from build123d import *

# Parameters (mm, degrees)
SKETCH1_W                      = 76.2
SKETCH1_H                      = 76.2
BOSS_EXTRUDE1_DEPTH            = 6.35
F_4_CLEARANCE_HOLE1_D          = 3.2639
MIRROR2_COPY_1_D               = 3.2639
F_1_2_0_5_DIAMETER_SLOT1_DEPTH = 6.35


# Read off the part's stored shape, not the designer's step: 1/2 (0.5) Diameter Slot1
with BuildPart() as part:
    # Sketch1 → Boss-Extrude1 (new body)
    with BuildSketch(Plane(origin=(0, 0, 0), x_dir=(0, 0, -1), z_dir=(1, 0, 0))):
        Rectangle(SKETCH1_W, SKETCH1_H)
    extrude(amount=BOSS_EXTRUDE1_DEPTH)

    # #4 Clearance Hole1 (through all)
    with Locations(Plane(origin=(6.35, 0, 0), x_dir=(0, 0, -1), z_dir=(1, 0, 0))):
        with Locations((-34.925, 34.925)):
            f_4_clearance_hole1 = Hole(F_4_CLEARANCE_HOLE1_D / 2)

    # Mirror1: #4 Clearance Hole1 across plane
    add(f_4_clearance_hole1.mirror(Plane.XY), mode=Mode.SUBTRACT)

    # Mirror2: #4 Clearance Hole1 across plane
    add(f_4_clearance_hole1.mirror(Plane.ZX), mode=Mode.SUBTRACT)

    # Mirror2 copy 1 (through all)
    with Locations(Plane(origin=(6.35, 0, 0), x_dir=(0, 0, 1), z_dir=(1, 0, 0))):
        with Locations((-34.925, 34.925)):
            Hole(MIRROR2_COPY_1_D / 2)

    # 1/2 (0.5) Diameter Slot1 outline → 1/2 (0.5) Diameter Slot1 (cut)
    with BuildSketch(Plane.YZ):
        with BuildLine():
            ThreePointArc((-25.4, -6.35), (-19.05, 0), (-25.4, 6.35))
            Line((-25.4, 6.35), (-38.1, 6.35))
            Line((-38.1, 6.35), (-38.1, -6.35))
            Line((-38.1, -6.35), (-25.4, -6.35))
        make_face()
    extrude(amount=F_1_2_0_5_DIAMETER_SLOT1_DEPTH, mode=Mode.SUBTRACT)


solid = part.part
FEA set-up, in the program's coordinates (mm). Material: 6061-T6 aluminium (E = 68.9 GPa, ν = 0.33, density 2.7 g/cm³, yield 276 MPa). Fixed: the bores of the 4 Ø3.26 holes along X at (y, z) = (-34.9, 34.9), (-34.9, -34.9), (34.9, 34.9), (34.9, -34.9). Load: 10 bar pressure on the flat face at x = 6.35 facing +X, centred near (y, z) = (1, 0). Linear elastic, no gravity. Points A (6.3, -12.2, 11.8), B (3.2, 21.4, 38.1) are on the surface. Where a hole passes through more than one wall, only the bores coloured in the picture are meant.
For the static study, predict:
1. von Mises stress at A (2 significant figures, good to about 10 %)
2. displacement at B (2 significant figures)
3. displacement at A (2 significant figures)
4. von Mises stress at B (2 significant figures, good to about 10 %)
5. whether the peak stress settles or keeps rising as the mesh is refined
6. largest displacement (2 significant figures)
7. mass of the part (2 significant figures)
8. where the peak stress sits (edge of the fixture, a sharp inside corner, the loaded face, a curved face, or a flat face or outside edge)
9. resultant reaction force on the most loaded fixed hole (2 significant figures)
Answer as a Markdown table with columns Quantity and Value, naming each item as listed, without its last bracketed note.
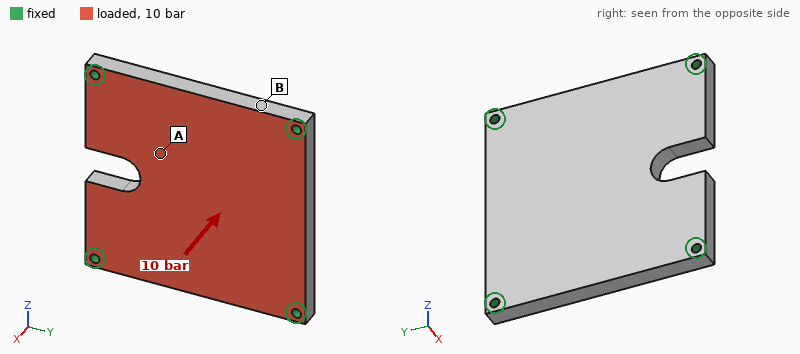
| Quantity | Value |
|---|---|
| von Mises stress at A | 43 MPa |
| displacement at B | 0.028 mm |
| displacement at A | 0.14 mm |
| von Mises stress at B | 22 MPa |
| whether the peak stress settles or keeps rising as the mesh is refined | keeps rising |
| largest displacement | 0.15 mm |
| mass of the part | 95 g |
| where the peak stress sits | edge of the fixture |
| resultant reaction force on the most loaded fixed hole | 1.4 kN |
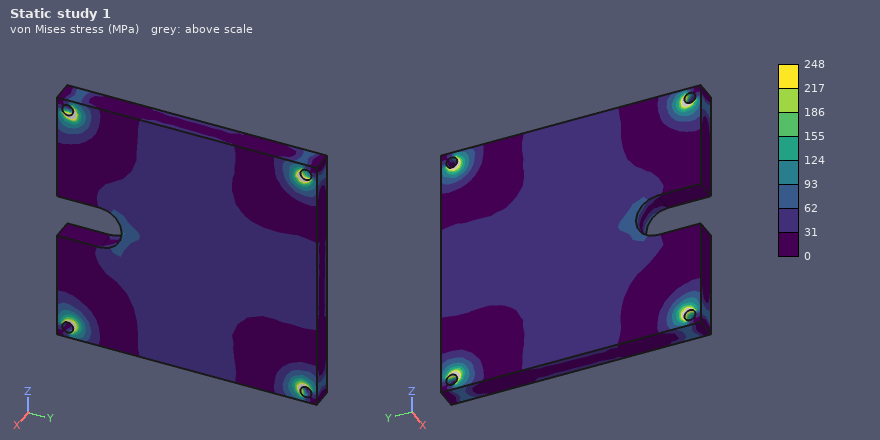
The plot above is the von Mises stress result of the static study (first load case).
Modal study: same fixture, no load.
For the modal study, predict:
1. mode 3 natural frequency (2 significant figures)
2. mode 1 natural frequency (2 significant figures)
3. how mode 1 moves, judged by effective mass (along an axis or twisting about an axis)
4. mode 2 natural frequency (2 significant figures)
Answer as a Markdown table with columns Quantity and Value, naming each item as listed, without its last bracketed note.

| Quantity | Value |
|---|---|
| mode 3 natural frequency | 6800 Hz |
| mode 1 natural frequency | 3700 Hz |
| how mode 1 moves, judged by effective mass | along X |
| mode 2 natural frequency | 6600 Hz |
